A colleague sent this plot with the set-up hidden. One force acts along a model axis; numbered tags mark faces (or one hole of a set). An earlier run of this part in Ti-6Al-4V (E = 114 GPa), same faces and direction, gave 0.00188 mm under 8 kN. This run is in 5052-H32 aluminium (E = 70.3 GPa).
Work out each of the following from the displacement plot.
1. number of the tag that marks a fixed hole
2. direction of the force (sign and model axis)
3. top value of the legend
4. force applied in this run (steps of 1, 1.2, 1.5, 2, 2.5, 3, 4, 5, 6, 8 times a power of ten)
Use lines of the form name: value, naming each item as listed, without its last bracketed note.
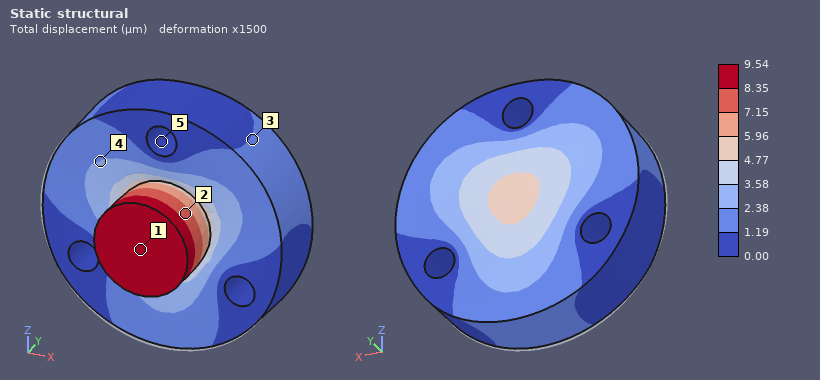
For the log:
number of the tag that marks a fixed hole: 5
direction of the force: +Y
top value of the legend: 9.54 µm
force applied in this run: 25 kN
